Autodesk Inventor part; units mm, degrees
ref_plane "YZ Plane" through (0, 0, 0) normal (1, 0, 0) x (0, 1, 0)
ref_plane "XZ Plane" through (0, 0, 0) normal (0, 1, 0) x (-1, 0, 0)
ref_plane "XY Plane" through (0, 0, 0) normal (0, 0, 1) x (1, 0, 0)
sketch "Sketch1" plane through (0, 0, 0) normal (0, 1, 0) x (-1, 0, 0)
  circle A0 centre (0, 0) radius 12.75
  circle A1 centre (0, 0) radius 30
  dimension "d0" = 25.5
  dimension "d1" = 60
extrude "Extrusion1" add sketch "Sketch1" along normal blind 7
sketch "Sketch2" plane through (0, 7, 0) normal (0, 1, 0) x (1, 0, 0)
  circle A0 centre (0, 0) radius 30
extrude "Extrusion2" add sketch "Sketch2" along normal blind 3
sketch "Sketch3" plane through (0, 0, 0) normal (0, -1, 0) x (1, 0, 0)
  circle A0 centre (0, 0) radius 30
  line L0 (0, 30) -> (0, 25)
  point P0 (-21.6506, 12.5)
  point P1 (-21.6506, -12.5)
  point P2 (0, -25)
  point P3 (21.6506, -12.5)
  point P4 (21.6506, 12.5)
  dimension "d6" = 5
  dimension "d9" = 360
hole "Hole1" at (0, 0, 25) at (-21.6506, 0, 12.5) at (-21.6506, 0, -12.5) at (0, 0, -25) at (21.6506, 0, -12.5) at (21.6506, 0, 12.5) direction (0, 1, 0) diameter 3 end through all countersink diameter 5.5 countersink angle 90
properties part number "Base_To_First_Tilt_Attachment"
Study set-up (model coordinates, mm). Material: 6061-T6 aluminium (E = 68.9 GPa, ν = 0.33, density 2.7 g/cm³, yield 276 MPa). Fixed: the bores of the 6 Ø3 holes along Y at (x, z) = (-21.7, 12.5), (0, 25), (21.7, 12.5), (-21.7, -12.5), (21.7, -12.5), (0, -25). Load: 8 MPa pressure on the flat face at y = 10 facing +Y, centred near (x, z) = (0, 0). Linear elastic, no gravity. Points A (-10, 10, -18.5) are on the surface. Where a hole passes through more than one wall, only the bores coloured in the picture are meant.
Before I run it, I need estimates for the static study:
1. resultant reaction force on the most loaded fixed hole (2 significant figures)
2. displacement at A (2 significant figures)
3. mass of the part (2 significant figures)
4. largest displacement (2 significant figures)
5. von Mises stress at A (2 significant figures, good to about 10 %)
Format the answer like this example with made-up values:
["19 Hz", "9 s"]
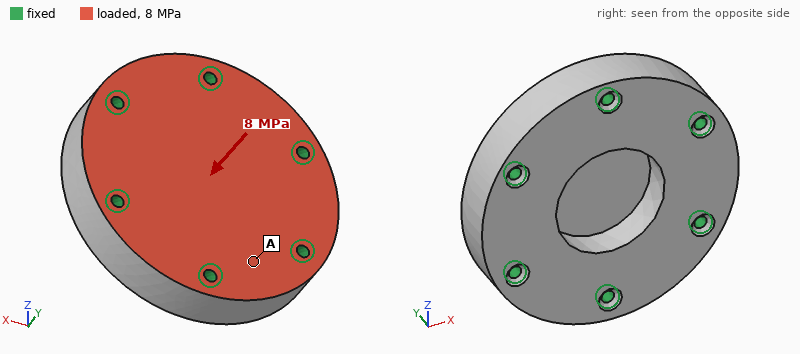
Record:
["3.8 kN", "9.8 µm", "65 g", "55 µm", "26 MPa"]
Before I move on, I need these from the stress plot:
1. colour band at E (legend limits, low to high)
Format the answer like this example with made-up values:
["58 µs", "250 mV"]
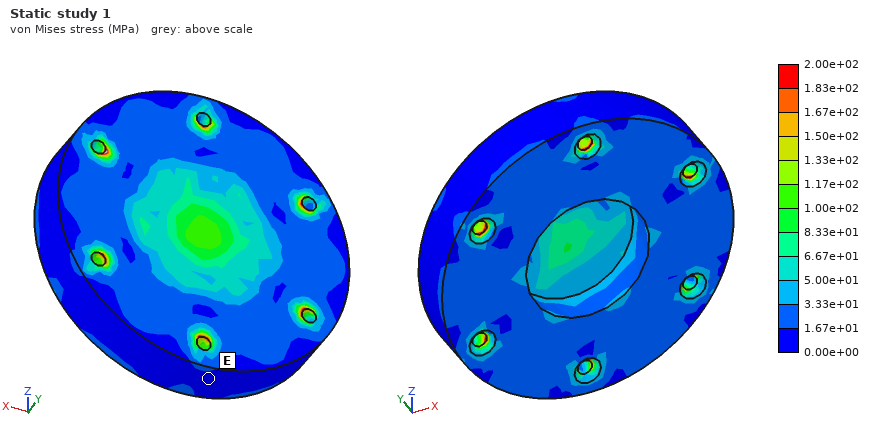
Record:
["0.00e+00 to 1.67e+01 MPa"]
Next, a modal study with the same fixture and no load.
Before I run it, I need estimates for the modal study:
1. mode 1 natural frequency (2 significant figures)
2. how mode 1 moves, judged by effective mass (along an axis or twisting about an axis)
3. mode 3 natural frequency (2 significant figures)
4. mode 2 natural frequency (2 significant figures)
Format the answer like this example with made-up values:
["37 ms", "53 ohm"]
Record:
["25 kHz", "along Y", "35 kHz", "35 kHz"]
